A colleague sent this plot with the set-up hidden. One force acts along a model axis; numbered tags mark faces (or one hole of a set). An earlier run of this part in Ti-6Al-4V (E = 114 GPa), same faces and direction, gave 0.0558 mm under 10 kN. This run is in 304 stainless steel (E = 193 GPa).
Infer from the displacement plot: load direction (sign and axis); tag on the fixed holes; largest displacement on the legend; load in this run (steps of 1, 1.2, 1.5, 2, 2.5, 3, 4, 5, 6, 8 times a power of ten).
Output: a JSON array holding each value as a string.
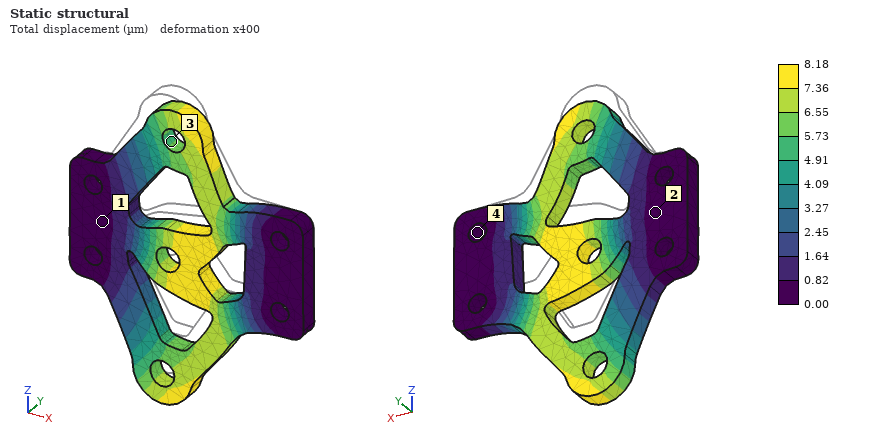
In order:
["-Z", "4", "8.18 µm", "2.5 kN"]
